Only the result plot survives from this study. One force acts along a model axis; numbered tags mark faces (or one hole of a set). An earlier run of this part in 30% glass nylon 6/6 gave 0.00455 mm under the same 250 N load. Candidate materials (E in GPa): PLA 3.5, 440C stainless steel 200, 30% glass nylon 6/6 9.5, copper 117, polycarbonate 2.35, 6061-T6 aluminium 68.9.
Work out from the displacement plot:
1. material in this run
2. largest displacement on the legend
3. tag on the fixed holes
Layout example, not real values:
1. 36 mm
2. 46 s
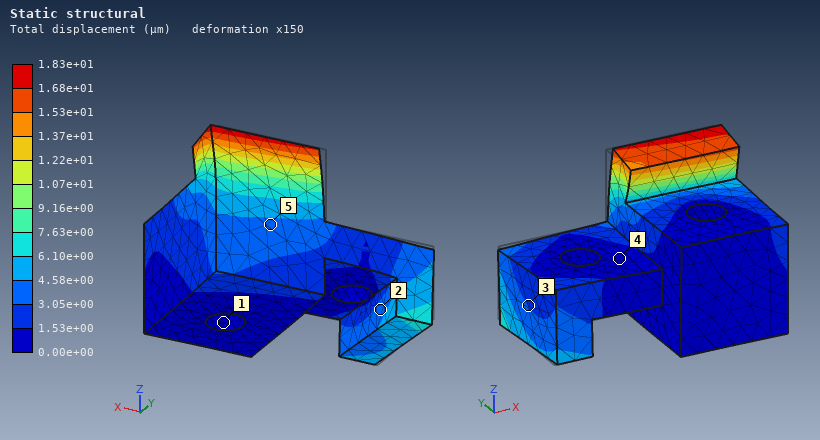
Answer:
1. polycarbonate
2. 1.83e+01 µm
3. 1
